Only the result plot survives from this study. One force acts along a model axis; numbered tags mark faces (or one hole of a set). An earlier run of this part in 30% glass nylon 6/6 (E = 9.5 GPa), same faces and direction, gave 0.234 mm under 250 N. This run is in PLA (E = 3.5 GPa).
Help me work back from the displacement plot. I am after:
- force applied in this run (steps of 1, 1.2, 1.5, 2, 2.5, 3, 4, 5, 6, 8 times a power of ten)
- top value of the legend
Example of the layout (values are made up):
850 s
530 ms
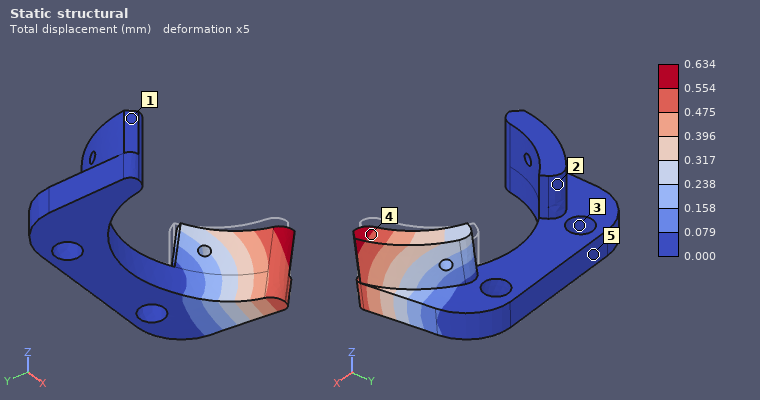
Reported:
250 N
0.634 mm
